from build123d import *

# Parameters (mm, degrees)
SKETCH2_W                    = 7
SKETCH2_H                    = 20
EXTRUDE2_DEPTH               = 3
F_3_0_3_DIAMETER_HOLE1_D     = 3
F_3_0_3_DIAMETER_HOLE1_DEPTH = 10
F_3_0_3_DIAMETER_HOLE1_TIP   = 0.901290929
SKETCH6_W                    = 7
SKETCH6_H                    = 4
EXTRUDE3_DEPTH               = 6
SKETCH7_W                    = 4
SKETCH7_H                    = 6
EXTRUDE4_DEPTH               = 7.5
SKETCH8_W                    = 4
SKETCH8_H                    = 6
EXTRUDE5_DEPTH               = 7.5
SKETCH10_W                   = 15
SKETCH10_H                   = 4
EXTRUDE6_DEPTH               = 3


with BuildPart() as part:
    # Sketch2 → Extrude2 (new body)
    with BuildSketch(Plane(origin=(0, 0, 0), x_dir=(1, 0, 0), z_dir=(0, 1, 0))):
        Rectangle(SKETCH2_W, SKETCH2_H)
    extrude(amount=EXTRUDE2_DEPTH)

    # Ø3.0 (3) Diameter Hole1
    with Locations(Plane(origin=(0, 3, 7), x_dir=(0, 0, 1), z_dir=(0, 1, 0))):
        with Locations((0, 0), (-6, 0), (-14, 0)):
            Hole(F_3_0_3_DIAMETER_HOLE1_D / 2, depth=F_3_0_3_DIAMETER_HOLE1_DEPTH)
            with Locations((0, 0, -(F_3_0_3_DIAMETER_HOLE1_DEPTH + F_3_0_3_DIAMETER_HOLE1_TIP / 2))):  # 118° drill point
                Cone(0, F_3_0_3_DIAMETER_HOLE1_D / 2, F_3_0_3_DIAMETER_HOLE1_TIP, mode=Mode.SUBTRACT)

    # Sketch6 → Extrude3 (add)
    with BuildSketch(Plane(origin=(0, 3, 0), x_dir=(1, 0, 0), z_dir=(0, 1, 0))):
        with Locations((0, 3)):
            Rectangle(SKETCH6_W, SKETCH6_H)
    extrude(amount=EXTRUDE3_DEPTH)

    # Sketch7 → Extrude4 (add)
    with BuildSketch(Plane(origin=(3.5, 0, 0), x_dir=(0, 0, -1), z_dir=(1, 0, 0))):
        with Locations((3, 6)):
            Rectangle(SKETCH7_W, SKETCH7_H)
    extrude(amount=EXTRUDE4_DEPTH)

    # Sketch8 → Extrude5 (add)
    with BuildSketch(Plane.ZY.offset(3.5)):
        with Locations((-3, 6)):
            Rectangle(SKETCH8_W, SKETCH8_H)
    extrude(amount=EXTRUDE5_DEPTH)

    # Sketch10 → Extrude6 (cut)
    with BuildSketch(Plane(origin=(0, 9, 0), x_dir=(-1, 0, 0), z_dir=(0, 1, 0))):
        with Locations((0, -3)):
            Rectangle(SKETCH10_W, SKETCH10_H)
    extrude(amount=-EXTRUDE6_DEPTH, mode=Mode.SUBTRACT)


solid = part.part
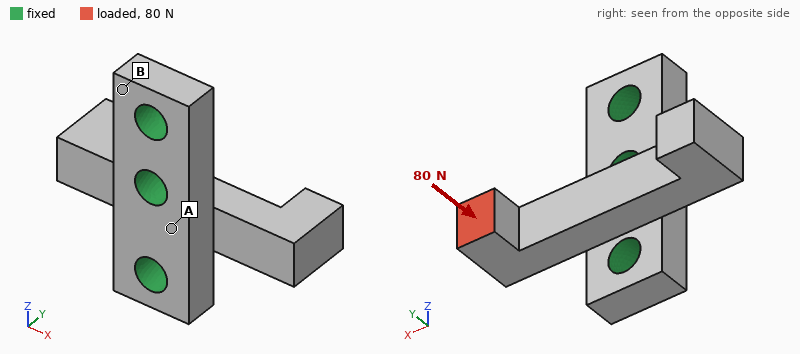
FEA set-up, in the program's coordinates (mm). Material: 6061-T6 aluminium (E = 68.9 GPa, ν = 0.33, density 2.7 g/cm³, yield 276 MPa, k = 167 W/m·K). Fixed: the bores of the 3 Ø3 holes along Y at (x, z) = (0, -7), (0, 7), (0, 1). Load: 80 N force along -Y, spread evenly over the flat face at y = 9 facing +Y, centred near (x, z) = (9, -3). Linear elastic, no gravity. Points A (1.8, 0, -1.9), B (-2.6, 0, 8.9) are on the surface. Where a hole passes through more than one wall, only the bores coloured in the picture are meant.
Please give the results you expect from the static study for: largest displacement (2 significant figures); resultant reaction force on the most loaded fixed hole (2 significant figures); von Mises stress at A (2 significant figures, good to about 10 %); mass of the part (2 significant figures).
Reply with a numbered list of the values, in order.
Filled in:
1. 36 µm
2. 53 N
3. 12 MPa
4. 1.9 g
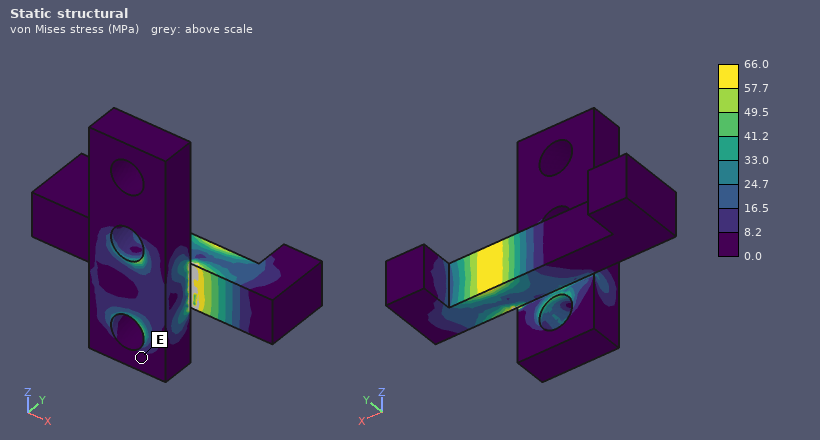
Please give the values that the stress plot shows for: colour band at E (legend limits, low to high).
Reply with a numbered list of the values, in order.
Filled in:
1. 0.0 to 8.2 MPa
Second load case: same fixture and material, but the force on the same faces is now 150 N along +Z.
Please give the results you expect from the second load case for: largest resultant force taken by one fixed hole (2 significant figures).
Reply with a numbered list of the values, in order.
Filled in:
1. 260 N
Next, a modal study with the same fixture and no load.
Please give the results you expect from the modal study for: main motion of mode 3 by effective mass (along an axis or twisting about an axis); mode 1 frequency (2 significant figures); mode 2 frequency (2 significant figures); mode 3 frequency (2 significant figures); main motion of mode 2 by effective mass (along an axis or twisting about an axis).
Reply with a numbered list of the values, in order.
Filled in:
1. twisting about Y
2. 15 kHz
3. 19 kHz
4. 20 kHz
5. along Y
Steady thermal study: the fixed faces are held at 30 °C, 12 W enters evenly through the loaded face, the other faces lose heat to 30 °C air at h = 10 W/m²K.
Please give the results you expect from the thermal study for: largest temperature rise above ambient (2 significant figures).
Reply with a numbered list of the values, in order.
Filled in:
1. 66 K
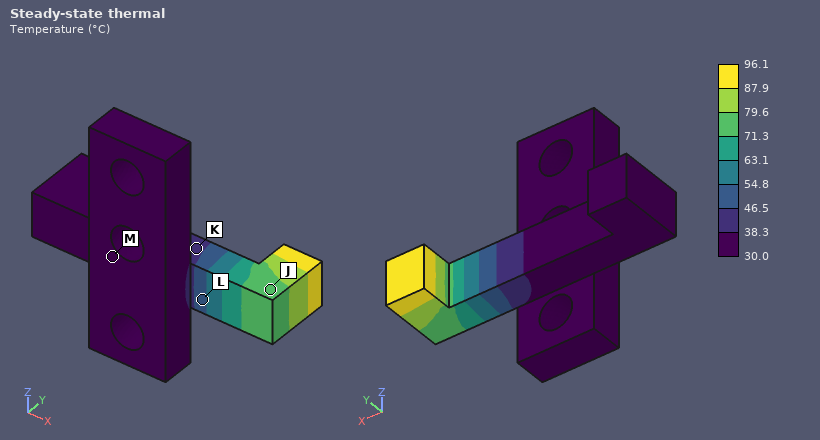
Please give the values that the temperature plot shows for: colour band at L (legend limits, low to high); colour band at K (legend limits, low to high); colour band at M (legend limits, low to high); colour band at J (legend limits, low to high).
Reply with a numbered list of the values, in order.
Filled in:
1. 46.5 to 54.8 °C
2. 38.3 to 46.5 °C
3. 30.0 to 38.3 °C
4. 71.3 to 79.6 °C
